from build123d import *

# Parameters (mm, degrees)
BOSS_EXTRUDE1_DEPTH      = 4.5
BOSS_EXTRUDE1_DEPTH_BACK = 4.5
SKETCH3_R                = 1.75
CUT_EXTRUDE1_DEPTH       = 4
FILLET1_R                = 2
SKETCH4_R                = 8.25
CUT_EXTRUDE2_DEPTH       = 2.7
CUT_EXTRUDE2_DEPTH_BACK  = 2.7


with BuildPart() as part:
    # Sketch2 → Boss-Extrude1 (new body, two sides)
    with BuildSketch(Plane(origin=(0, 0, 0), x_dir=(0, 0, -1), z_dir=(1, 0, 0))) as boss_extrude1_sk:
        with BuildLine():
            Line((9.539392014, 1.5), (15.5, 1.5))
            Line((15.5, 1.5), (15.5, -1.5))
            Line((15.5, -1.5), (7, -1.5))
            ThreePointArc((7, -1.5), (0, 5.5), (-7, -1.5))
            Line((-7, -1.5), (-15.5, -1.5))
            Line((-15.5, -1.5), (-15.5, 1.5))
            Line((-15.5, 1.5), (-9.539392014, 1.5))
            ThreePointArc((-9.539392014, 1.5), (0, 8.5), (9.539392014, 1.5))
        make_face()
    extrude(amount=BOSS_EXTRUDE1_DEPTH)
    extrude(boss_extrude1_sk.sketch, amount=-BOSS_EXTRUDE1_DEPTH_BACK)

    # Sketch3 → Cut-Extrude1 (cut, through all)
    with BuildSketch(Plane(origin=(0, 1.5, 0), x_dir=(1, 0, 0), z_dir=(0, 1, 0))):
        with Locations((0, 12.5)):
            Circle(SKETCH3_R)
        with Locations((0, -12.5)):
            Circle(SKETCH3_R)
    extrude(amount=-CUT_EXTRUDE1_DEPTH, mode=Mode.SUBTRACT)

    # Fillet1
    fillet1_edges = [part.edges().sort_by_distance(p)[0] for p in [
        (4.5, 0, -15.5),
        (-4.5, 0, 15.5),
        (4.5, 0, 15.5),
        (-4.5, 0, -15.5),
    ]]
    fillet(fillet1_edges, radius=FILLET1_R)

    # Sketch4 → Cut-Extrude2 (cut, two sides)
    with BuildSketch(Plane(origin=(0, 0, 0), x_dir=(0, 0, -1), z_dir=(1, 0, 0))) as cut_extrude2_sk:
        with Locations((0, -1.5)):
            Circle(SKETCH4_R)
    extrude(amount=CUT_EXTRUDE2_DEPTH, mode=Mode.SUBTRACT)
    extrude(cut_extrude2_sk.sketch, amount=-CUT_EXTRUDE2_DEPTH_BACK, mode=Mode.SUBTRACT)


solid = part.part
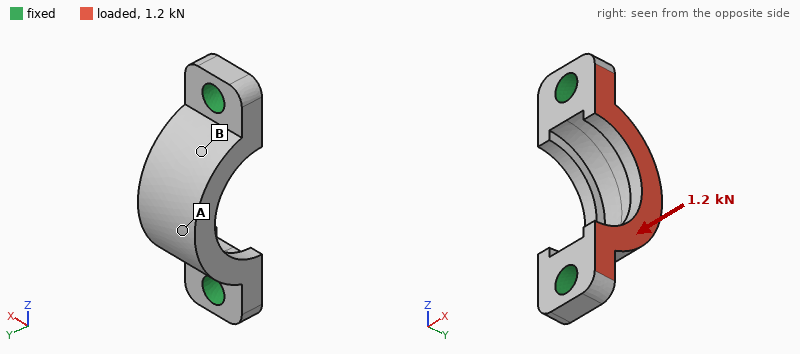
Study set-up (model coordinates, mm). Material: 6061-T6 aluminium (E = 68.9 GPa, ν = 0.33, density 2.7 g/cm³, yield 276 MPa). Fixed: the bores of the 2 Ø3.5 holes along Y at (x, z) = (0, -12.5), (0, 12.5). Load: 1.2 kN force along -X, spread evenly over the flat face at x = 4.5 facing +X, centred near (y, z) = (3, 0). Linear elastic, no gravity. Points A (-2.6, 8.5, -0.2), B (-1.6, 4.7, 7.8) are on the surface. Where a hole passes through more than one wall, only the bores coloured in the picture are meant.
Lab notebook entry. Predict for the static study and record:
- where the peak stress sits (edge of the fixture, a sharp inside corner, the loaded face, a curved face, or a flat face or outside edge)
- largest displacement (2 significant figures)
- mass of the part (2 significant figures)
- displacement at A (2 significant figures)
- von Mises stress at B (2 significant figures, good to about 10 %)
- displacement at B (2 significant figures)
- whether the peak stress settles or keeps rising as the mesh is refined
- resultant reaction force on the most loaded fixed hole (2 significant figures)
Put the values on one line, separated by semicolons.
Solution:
edge of the fixture; 41 µm; 2.2 g; 39 µm; 45 MPa; 20 µm; keeps rising; 600 N
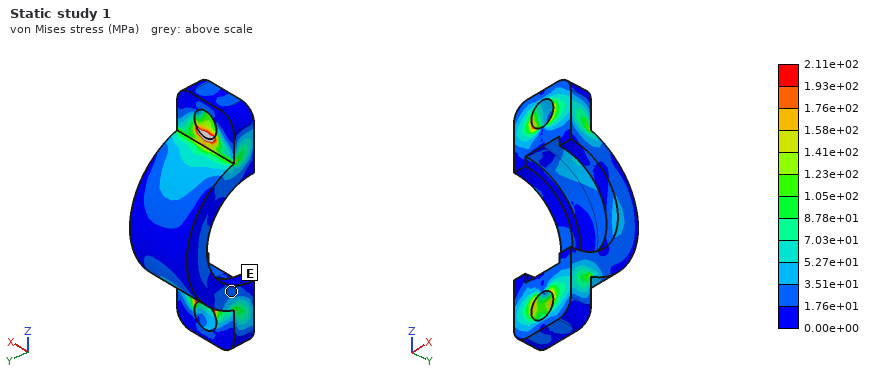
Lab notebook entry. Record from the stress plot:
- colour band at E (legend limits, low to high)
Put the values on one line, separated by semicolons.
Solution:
1.76e+01 to 3.51e+01 MPa
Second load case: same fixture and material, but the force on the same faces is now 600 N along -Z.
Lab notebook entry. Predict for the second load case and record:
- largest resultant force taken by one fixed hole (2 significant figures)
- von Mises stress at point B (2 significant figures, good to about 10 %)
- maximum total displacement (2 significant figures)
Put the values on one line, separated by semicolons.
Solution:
310 N; 14 MPa; 14 µm
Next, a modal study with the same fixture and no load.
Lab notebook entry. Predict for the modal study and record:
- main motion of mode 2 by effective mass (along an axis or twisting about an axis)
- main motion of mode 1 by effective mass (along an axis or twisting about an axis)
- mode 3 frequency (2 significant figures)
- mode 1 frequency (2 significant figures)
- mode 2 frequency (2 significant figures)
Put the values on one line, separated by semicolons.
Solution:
along Z; along X; 46 kHz; 22 kHz; 35 kHz
